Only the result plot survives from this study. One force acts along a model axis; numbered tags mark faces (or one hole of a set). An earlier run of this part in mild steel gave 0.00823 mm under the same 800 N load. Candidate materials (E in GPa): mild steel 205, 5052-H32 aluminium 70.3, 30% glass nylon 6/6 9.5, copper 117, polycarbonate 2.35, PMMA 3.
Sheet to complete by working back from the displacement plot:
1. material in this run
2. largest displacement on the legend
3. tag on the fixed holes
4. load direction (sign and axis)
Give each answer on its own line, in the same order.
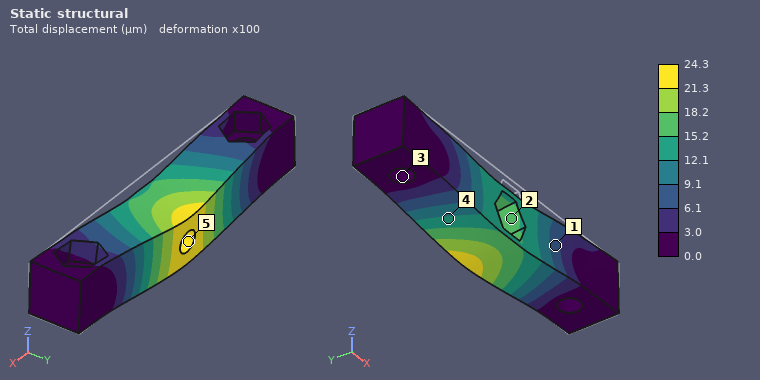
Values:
5052-H32 aluminium
24.3 µm
3
-Z
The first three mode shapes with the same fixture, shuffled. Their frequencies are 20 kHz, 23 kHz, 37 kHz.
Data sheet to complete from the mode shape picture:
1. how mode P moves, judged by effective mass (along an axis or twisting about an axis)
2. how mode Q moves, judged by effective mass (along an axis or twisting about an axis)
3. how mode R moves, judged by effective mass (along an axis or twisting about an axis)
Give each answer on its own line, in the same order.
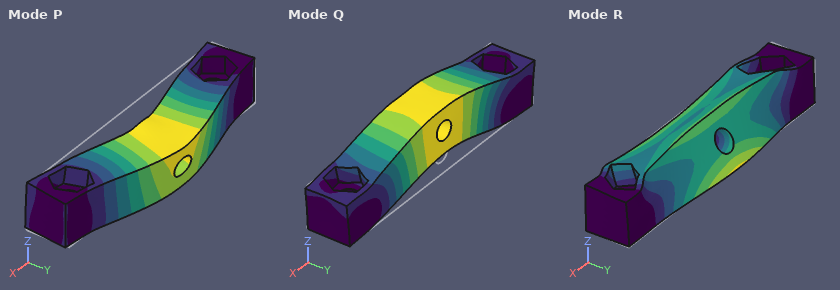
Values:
along Y
along Z
twisting about X
